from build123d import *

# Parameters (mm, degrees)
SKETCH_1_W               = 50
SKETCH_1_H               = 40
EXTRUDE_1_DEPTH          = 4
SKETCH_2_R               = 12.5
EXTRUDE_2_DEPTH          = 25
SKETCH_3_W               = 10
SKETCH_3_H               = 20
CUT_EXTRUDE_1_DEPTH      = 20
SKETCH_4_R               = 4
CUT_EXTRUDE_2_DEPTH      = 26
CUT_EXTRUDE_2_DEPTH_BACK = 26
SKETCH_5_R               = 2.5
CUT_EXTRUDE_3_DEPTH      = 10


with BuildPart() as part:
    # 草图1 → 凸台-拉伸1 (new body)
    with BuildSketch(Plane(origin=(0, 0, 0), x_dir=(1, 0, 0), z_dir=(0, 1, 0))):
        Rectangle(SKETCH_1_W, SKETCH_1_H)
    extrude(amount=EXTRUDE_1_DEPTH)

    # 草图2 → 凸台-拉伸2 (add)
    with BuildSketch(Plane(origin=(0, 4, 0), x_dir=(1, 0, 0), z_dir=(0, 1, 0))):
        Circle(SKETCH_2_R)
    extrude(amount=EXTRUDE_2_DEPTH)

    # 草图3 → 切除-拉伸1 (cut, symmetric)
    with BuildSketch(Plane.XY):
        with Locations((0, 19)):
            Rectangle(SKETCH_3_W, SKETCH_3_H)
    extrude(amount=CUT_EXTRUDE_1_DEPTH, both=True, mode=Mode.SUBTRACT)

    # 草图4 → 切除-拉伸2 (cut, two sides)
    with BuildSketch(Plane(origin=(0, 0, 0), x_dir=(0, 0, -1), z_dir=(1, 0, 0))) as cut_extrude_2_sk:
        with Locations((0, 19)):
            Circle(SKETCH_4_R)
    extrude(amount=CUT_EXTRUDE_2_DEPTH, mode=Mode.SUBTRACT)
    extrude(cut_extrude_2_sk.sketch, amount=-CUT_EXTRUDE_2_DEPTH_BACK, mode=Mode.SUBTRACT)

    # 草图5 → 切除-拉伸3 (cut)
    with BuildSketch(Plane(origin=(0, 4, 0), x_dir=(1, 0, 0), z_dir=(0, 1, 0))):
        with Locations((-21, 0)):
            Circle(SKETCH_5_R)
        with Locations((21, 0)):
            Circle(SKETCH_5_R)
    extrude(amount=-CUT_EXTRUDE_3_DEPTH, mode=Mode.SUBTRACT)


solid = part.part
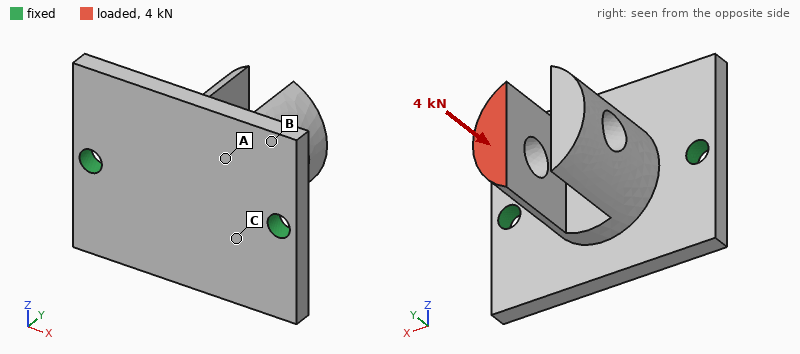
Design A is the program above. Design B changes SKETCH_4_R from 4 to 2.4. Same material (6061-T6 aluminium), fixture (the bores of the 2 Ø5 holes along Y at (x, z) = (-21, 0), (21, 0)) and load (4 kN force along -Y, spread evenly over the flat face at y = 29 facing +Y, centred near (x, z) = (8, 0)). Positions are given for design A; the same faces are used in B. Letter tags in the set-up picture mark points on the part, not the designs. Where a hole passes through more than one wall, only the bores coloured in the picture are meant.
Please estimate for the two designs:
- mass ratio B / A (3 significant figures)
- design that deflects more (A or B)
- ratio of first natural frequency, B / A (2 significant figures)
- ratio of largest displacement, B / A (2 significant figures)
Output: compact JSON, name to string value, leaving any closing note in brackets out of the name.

{"mass ratio B / A": "1.03", "design that deflects more": "A", "ratio of first natural frequency, B / A": "0.97", "ratio of largest displacement, B / A": "0.86"}
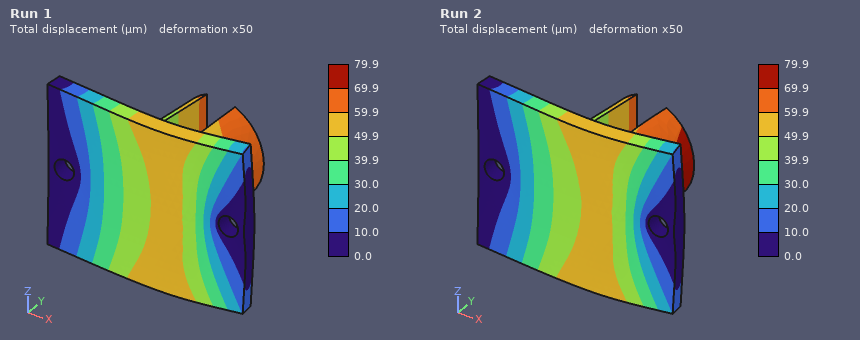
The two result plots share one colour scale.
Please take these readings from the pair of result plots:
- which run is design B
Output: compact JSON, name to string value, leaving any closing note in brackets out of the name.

{"which run is design B": "Run 1"}
